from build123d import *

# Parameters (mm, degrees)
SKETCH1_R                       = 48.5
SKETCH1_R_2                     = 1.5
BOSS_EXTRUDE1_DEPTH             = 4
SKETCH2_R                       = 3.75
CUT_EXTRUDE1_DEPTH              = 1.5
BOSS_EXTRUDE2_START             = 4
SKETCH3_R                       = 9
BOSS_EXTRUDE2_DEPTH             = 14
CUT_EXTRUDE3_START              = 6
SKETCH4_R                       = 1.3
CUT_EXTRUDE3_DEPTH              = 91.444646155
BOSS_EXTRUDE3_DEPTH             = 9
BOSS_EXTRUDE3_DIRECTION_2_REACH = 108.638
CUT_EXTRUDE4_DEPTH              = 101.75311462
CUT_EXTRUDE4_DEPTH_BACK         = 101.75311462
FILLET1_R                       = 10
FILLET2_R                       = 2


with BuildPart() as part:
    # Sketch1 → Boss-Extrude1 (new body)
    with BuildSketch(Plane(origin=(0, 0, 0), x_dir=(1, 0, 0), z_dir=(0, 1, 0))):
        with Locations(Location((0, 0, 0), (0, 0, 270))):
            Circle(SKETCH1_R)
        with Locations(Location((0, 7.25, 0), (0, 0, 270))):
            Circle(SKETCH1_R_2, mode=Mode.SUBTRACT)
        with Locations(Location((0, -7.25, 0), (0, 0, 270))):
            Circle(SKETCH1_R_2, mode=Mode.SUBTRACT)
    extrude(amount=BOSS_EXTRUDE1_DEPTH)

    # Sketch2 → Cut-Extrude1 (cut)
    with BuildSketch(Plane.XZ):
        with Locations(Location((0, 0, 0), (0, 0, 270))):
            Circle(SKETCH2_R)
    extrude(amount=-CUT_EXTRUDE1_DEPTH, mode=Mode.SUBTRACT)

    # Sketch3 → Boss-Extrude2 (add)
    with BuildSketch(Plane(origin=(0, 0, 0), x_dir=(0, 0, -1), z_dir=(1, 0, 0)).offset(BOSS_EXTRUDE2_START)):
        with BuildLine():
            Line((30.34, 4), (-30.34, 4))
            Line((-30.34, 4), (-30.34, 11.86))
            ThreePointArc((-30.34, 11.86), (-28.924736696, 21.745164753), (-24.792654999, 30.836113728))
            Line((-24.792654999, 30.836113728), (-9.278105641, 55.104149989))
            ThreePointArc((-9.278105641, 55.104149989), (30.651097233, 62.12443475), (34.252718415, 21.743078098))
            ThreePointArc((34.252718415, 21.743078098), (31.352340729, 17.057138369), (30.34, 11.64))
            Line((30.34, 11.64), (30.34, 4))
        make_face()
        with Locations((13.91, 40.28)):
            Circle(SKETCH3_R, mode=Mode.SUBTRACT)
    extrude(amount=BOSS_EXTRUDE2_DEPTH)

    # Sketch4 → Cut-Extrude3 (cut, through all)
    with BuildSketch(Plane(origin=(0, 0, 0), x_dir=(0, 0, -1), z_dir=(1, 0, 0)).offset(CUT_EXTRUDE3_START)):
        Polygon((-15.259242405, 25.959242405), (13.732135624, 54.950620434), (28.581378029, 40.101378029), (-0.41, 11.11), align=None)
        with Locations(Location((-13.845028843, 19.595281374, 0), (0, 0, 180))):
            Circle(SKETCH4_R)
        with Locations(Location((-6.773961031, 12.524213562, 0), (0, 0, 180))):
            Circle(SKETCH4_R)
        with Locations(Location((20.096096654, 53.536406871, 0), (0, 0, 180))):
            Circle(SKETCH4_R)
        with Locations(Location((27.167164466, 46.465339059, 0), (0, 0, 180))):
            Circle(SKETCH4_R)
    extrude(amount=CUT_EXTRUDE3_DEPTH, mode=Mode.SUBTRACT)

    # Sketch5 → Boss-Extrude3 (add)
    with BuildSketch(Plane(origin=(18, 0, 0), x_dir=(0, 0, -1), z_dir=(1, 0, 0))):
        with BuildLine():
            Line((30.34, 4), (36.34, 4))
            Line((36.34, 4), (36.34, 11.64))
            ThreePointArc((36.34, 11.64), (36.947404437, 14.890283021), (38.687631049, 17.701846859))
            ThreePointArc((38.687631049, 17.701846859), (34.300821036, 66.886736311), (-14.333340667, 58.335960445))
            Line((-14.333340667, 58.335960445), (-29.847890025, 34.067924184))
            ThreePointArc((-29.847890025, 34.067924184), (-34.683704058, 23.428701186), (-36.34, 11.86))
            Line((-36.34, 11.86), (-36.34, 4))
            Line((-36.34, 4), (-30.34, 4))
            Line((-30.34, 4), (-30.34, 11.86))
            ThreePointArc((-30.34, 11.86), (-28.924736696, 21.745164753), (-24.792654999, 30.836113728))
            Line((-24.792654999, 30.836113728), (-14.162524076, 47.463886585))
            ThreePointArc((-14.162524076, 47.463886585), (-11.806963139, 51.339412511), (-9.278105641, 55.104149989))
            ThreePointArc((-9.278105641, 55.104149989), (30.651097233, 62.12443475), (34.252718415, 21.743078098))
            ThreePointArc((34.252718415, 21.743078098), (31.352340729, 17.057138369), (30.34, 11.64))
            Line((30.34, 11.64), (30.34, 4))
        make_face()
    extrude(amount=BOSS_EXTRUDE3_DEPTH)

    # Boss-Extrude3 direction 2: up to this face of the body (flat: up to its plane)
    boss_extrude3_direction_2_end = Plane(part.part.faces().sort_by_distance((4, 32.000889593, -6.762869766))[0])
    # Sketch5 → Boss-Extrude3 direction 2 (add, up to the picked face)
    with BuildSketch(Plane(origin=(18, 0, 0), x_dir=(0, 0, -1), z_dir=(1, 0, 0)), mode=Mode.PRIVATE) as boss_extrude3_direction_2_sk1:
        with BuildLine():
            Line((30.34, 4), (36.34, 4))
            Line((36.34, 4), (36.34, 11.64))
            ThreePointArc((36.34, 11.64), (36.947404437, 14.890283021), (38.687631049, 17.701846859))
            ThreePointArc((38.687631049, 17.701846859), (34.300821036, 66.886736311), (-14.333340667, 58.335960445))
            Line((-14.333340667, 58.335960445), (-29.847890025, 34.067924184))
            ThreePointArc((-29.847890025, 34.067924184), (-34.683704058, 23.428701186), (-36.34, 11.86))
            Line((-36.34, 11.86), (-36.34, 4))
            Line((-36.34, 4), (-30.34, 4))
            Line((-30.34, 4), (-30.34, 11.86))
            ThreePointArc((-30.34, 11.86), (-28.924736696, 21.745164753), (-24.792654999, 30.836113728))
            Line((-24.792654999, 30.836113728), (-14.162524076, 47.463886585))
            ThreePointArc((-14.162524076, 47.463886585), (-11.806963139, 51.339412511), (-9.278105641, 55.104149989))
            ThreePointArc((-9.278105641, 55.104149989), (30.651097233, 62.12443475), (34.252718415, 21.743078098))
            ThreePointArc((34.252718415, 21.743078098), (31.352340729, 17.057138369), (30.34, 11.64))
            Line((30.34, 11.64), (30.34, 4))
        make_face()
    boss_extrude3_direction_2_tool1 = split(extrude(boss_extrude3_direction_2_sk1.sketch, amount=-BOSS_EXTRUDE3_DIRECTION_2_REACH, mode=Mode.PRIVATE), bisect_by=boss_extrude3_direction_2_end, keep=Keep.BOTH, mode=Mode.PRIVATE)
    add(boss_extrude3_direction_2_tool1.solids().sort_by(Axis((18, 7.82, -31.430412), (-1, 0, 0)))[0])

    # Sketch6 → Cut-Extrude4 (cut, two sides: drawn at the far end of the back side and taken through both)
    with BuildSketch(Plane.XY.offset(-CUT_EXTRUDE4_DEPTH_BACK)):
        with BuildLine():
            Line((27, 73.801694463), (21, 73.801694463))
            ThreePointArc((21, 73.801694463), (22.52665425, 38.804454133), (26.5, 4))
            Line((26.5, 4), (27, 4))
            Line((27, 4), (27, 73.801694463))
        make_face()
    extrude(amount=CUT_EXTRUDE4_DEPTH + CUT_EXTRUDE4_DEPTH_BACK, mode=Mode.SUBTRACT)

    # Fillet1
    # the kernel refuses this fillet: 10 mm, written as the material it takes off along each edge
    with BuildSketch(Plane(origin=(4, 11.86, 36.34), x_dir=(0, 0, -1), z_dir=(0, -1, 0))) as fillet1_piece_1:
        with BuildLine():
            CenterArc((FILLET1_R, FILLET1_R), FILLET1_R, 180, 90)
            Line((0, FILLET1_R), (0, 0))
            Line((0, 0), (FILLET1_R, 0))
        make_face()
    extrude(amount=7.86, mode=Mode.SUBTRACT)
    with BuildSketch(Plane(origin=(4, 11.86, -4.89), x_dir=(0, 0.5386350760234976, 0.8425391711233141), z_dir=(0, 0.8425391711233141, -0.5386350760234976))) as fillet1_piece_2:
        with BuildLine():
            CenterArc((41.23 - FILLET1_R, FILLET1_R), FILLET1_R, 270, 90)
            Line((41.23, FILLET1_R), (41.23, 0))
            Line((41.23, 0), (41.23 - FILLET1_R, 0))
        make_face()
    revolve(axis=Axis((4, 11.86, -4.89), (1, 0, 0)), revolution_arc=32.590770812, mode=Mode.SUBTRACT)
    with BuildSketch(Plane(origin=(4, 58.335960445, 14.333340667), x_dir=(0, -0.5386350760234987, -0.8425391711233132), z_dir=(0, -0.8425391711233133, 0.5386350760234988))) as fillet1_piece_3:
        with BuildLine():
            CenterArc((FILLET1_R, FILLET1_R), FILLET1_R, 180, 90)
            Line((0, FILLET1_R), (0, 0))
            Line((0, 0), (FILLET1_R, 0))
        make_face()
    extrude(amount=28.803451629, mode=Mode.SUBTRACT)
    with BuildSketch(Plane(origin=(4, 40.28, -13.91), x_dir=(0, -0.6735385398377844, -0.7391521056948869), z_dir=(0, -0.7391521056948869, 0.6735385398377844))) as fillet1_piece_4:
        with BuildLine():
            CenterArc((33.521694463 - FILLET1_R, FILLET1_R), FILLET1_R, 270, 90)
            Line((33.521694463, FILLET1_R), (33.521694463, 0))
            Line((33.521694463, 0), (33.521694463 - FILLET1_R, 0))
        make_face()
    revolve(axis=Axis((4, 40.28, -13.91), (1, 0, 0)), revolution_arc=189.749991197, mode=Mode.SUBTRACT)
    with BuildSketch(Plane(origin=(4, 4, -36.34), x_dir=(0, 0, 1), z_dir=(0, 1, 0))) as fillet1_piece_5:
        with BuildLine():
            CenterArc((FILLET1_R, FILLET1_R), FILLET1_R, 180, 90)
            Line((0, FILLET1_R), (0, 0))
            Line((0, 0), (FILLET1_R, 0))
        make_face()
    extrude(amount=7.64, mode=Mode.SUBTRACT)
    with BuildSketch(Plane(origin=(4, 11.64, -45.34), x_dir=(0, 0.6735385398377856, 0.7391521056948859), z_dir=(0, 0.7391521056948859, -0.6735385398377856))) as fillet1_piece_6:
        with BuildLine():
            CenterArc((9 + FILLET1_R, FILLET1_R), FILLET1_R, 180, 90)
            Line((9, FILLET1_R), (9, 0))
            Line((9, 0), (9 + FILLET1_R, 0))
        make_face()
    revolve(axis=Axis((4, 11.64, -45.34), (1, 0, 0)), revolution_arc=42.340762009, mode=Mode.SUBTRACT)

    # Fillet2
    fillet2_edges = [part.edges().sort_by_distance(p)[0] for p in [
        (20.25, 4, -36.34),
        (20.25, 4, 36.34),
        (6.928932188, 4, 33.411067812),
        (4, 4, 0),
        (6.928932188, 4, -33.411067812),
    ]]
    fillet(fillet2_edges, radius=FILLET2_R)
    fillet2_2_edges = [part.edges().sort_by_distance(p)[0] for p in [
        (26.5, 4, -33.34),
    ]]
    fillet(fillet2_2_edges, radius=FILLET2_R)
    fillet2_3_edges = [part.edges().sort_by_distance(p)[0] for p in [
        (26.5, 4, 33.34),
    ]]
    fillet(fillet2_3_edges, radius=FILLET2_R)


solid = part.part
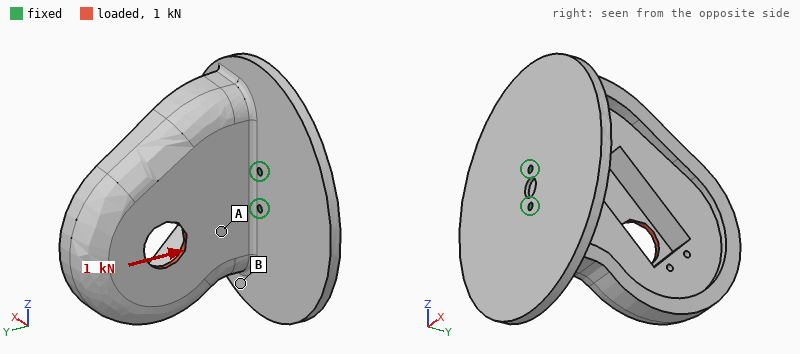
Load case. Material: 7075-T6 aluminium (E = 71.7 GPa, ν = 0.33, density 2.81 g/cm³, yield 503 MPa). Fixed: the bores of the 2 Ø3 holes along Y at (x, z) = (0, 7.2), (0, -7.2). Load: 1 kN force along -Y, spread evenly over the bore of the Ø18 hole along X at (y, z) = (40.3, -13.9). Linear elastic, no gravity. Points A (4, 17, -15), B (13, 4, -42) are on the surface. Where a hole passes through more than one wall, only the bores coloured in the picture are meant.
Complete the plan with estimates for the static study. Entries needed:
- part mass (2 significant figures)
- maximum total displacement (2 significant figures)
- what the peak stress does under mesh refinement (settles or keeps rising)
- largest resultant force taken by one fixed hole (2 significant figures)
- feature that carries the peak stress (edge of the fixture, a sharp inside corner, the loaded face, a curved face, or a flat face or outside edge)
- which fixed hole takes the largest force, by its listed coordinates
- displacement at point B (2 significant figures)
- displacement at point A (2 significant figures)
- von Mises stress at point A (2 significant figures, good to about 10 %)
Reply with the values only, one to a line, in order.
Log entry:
230 g
97 µm
keeps rising
1.2 kN
edge of the fixture
(0, -7.2)
51 µm
28 µm
8.1 MPa
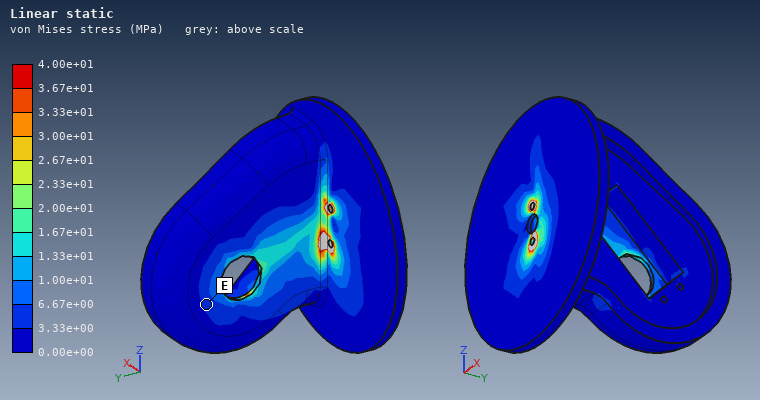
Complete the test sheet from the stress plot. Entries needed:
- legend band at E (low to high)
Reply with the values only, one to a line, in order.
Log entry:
3.33e+00 to 6.67e+00 MPa
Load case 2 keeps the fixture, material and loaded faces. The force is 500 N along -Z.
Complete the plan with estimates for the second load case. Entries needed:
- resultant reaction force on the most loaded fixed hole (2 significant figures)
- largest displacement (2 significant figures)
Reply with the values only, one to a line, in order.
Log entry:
1.1 kN
84 µm
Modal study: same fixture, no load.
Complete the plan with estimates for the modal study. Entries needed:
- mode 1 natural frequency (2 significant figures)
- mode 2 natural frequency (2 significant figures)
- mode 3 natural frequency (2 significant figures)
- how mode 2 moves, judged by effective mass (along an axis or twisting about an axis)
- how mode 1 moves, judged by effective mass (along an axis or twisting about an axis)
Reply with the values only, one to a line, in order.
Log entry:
510 Hz
1100 Hz
1600 Hz
along Z
along X
